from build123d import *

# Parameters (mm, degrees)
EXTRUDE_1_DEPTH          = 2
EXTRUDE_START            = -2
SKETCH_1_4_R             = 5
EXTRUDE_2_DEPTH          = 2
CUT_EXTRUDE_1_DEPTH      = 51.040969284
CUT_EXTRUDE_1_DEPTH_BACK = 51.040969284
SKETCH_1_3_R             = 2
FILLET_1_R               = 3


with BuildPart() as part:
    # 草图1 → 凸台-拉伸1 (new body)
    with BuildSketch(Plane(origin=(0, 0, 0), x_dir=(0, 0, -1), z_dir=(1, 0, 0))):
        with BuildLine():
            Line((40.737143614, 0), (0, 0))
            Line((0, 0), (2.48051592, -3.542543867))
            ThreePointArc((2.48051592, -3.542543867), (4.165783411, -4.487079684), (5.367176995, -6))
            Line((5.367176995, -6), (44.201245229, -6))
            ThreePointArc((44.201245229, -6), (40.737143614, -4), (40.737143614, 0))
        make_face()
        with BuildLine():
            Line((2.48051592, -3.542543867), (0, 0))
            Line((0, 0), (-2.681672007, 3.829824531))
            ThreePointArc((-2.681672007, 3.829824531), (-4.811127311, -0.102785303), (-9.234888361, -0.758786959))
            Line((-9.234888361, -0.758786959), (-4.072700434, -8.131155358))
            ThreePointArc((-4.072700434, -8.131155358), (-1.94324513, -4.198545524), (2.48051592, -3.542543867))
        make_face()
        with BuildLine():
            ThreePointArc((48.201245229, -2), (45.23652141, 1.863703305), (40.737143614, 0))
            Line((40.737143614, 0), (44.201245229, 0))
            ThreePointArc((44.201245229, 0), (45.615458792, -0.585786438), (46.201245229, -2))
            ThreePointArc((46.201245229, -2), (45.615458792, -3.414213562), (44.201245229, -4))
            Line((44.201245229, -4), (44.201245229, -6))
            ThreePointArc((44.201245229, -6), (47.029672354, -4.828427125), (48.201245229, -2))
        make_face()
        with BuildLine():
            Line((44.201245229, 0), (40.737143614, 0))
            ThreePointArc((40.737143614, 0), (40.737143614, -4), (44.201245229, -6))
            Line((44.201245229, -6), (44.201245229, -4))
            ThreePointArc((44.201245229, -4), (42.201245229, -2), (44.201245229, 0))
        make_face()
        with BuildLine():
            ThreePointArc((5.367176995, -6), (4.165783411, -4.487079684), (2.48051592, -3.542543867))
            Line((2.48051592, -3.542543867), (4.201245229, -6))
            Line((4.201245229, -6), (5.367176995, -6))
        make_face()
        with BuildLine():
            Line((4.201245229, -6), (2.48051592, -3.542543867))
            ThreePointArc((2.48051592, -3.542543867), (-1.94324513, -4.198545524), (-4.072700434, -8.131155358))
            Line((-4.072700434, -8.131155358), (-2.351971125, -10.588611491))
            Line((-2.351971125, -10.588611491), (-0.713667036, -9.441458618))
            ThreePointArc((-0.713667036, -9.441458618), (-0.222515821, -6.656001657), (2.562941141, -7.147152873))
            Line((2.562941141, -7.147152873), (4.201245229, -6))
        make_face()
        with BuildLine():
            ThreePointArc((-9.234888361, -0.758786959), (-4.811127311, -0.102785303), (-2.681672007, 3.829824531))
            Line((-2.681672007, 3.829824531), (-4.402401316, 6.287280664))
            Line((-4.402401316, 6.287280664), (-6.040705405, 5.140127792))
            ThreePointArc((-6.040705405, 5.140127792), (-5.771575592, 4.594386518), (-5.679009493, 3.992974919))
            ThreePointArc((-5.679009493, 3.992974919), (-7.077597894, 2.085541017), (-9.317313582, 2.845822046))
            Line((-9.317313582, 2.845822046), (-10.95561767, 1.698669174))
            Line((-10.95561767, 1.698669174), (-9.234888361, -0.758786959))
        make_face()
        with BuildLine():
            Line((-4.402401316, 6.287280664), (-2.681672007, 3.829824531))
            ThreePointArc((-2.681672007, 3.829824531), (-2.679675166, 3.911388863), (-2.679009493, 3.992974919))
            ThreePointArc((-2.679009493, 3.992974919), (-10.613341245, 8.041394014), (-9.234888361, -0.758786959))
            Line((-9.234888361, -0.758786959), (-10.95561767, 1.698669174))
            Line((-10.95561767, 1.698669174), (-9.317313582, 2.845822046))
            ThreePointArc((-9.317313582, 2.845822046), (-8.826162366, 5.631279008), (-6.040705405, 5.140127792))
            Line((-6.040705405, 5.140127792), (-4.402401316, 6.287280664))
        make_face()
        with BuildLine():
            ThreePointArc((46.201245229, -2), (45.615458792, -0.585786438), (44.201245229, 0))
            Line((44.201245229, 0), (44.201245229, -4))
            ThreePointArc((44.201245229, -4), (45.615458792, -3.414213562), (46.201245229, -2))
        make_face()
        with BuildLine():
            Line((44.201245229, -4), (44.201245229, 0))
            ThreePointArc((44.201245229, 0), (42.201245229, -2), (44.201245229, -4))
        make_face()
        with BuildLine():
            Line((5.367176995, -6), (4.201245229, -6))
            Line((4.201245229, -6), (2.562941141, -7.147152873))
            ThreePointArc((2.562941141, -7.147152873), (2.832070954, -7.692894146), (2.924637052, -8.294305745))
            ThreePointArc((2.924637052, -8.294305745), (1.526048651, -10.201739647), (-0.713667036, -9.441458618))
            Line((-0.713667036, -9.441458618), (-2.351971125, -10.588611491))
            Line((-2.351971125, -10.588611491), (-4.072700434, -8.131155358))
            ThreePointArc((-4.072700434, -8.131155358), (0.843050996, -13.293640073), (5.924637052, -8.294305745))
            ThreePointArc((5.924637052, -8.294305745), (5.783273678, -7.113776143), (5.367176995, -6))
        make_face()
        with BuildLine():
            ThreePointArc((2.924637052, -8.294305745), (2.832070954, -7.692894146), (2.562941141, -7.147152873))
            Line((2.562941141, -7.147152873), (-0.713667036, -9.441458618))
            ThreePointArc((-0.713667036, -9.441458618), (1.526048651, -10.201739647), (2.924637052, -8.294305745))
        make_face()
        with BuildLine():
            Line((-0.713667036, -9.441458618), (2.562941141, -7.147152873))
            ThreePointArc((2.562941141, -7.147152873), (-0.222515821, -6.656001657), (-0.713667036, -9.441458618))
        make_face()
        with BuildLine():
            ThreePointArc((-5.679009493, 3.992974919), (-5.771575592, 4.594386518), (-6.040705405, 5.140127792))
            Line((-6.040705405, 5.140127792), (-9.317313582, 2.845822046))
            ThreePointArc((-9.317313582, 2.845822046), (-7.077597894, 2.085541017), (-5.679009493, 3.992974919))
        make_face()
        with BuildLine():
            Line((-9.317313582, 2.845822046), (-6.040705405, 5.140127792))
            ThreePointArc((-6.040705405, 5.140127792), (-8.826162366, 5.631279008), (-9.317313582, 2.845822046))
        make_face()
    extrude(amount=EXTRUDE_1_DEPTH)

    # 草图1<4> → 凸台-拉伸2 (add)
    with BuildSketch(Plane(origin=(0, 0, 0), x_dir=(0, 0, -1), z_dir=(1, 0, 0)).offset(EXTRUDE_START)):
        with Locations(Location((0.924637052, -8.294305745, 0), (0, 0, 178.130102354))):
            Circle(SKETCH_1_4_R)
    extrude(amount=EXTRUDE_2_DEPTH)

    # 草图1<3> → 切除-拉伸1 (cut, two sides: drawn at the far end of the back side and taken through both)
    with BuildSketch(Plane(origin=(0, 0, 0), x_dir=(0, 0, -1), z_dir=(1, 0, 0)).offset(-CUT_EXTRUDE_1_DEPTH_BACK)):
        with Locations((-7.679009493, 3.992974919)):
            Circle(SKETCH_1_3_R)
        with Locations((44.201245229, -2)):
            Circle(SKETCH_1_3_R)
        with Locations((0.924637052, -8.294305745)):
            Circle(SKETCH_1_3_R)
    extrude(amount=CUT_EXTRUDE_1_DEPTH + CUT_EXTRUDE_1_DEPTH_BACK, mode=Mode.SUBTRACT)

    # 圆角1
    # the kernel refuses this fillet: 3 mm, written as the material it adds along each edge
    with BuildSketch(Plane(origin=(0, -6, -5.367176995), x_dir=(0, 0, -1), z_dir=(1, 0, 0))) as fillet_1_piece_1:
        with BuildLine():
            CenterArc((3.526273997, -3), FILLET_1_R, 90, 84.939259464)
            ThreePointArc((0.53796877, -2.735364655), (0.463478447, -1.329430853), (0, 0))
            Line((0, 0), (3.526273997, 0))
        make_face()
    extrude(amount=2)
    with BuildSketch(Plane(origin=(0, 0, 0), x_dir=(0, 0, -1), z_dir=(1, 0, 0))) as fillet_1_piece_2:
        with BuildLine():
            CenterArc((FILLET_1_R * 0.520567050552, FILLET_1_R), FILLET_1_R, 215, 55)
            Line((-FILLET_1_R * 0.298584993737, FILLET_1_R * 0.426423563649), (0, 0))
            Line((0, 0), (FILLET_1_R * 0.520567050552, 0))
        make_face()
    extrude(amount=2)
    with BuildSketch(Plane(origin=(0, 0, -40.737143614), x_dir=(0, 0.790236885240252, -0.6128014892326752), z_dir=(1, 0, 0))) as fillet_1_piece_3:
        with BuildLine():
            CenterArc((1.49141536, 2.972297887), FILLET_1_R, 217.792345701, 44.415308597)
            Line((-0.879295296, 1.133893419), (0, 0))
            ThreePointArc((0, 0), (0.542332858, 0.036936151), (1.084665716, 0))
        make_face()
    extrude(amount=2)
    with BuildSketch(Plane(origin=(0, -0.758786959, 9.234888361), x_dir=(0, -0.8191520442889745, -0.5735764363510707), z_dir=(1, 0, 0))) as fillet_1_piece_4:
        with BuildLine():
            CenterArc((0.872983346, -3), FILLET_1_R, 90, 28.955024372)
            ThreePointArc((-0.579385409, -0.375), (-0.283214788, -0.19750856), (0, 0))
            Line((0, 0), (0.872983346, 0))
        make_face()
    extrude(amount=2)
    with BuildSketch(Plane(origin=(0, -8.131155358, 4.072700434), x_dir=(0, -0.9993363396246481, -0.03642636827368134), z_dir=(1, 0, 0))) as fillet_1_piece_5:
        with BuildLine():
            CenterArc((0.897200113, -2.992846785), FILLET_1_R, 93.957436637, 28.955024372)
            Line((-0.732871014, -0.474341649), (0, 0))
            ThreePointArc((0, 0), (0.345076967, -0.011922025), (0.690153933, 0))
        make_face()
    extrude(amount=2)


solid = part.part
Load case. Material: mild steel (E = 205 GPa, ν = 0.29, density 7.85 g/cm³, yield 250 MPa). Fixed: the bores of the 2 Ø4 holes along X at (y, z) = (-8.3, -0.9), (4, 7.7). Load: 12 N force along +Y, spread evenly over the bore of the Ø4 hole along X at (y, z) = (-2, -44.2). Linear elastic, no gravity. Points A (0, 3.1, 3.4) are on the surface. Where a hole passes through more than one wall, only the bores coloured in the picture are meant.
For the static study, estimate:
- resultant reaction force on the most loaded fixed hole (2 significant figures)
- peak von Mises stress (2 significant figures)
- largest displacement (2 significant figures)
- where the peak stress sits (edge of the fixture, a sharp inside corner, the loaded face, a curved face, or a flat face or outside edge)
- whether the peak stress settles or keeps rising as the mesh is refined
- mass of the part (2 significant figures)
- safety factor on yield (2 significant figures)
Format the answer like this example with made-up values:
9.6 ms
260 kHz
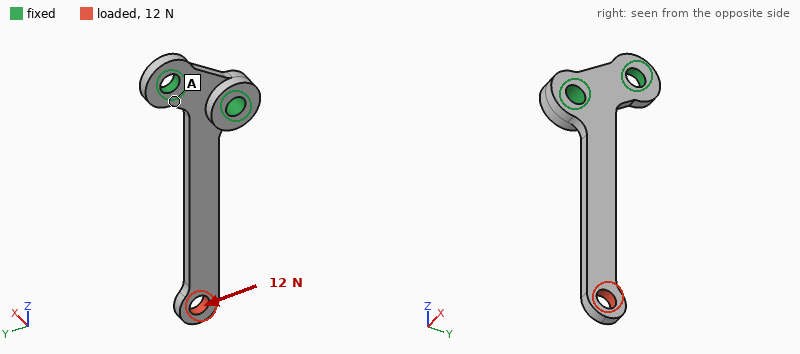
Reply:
30 N
49 MPa
41 µm
a curved face
settles
8.1 g
5.1
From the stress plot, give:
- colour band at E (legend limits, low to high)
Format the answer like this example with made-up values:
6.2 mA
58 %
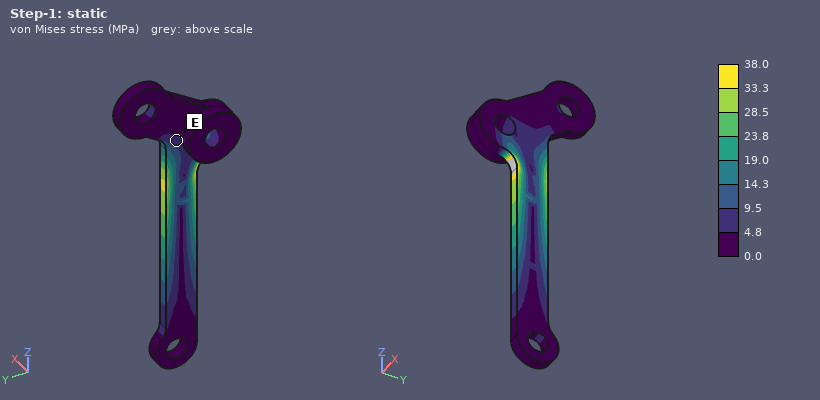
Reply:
4.8 to 9.5 MPa
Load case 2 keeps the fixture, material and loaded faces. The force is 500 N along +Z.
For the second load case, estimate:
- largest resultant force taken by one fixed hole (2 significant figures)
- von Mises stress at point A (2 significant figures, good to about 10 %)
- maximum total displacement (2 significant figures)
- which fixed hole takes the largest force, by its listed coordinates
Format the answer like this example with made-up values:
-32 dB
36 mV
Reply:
330 N
12 MPa
81 µm
(-8.3, -0.9)
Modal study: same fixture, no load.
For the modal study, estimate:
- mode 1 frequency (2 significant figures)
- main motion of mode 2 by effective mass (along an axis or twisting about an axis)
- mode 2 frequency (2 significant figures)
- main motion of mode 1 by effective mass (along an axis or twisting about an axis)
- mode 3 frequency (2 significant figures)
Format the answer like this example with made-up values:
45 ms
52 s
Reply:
880 Hz
along Y
2600 Hz
along X
5300 Hz
